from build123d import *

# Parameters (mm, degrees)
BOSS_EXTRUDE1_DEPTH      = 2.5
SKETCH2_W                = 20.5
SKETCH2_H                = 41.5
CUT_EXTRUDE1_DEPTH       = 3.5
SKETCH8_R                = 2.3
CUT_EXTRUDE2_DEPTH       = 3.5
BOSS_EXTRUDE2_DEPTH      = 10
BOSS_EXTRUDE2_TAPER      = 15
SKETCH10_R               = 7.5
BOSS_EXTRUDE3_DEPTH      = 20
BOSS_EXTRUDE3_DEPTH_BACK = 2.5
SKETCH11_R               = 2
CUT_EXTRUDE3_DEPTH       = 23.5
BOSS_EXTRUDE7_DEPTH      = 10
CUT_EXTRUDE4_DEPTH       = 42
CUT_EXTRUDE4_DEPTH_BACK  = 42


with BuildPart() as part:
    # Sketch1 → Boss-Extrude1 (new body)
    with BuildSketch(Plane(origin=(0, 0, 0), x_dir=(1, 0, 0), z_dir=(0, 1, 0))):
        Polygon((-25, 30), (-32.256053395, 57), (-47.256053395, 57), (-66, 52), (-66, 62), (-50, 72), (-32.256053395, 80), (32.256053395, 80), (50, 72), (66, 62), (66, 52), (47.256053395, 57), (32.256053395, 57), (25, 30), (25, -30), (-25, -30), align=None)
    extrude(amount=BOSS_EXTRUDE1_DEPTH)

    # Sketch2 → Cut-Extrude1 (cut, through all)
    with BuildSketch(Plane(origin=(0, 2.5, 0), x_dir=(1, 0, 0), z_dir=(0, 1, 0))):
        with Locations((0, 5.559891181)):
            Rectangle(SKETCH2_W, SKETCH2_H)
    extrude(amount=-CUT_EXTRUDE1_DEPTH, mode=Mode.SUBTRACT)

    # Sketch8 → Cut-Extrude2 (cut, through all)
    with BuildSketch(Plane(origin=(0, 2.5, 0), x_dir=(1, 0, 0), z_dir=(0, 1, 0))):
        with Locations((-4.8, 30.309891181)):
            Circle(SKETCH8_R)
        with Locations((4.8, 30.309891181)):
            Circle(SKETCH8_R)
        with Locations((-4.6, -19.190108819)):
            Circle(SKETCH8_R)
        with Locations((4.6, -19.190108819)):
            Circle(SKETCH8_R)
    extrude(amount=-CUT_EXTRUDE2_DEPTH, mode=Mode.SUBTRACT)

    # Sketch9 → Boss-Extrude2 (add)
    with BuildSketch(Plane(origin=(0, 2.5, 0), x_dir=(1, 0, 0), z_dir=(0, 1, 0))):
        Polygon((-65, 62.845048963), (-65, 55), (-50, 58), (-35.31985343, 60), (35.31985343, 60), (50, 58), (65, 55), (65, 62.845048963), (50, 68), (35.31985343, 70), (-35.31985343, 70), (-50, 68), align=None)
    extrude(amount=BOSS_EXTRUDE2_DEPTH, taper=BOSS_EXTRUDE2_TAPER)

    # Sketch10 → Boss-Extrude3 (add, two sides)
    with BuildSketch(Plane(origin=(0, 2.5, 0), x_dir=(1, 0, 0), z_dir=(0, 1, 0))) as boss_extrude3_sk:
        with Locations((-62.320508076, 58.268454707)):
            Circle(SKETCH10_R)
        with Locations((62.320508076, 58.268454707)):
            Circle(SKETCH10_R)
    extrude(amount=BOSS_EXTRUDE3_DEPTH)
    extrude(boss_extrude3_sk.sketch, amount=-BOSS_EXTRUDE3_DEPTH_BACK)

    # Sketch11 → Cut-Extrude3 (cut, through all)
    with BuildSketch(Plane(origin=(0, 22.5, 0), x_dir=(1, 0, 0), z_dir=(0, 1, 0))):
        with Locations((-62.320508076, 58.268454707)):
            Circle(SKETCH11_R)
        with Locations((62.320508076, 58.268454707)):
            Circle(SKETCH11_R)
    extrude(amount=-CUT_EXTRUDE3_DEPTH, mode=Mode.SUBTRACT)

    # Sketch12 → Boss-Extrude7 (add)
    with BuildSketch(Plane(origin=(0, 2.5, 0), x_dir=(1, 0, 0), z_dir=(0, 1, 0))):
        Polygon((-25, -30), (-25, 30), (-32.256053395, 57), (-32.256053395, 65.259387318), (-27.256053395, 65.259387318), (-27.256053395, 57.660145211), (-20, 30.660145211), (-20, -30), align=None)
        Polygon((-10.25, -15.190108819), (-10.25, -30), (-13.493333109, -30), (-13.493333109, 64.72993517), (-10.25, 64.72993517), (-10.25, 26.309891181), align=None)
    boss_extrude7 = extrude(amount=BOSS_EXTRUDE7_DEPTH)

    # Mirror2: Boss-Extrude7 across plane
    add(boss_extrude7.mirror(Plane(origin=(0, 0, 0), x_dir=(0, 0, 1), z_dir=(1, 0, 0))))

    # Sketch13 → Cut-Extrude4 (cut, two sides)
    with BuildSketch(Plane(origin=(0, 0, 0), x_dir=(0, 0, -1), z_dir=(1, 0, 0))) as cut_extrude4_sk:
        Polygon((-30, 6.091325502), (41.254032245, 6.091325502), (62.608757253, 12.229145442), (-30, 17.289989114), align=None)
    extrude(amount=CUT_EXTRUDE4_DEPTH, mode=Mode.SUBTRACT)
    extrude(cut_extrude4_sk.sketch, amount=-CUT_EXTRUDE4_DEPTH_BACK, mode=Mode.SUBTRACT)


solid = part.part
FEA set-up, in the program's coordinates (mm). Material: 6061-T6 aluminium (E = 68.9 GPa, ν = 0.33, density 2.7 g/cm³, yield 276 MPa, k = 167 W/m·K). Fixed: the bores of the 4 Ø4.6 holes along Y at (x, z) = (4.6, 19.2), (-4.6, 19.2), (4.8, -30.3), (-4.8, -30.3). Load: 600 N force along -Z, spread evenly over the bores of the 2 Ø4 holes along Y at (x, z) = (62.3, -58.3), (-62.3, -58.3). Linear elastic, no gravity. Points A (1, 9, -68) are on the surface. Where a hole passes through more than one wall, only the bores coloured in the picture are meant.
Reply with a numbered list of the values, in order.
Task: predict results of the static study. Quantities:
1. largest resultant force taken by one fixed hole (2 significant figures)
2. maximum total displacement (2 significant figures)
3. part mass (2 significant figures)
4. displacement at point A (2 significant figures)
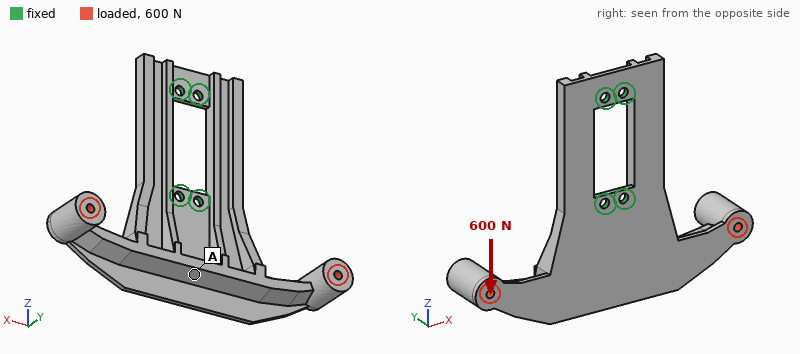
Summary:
1. 210 N
2. 0.24 mm
3. 99 g
4. 0.14 mm
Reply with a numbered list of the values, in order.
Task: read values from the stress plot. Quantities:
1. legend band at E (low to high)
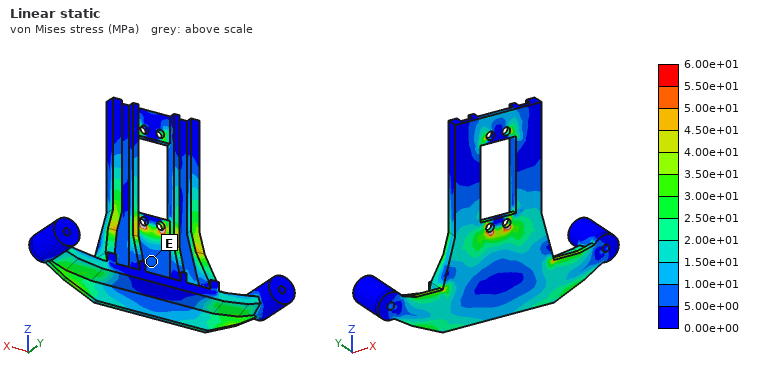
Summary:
1. 5.00e+00 to 1.00e+01 MPa
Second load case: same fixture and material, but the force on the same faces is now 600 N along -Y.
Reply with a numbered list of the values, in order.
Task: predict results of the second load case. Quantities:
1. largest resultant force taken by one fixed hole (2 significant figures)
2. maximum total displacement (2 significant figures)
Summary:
1. 510 N
2. 0.60 mm
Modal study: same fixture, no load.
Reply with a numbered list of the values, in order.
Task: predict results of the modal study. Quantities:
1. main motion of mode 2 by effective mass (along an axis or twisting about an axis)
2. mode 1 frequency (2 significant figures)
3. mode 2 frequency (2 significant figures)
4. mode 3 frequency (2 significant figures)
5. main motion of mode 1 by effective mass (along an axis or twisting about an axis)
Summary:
1. along Y
2. 440 Hz
3. 710 Hz
4. 2100 Hz
5. twisting about Z
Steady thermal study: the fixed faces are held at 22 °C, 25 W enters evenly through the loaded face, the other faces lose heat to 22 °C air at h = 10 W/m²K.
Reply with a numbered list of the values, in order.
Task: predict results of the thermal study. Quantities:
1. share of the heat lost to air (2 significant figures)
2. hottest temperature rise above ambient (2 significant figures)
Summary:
1. 17 %
2. 49 K
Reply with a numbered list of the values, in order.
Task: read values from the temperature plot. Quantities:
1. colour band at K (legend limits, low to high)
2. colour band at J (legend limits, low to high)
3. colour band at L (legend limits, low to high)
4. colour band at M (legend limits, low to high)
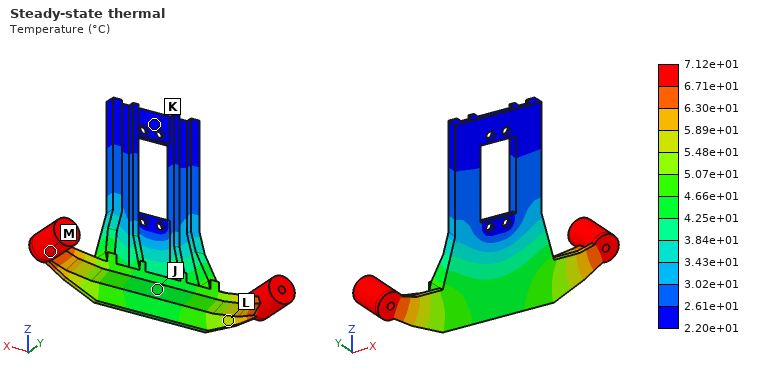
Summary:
1. 2.20e+01 to 2.61e+01 °C
2. 4.25e+01 to 4.66e+01 °C
3. 5.48e+01 to 5.89e+01 °C
4. 6.71e+01 to 7.12e+01 °C
